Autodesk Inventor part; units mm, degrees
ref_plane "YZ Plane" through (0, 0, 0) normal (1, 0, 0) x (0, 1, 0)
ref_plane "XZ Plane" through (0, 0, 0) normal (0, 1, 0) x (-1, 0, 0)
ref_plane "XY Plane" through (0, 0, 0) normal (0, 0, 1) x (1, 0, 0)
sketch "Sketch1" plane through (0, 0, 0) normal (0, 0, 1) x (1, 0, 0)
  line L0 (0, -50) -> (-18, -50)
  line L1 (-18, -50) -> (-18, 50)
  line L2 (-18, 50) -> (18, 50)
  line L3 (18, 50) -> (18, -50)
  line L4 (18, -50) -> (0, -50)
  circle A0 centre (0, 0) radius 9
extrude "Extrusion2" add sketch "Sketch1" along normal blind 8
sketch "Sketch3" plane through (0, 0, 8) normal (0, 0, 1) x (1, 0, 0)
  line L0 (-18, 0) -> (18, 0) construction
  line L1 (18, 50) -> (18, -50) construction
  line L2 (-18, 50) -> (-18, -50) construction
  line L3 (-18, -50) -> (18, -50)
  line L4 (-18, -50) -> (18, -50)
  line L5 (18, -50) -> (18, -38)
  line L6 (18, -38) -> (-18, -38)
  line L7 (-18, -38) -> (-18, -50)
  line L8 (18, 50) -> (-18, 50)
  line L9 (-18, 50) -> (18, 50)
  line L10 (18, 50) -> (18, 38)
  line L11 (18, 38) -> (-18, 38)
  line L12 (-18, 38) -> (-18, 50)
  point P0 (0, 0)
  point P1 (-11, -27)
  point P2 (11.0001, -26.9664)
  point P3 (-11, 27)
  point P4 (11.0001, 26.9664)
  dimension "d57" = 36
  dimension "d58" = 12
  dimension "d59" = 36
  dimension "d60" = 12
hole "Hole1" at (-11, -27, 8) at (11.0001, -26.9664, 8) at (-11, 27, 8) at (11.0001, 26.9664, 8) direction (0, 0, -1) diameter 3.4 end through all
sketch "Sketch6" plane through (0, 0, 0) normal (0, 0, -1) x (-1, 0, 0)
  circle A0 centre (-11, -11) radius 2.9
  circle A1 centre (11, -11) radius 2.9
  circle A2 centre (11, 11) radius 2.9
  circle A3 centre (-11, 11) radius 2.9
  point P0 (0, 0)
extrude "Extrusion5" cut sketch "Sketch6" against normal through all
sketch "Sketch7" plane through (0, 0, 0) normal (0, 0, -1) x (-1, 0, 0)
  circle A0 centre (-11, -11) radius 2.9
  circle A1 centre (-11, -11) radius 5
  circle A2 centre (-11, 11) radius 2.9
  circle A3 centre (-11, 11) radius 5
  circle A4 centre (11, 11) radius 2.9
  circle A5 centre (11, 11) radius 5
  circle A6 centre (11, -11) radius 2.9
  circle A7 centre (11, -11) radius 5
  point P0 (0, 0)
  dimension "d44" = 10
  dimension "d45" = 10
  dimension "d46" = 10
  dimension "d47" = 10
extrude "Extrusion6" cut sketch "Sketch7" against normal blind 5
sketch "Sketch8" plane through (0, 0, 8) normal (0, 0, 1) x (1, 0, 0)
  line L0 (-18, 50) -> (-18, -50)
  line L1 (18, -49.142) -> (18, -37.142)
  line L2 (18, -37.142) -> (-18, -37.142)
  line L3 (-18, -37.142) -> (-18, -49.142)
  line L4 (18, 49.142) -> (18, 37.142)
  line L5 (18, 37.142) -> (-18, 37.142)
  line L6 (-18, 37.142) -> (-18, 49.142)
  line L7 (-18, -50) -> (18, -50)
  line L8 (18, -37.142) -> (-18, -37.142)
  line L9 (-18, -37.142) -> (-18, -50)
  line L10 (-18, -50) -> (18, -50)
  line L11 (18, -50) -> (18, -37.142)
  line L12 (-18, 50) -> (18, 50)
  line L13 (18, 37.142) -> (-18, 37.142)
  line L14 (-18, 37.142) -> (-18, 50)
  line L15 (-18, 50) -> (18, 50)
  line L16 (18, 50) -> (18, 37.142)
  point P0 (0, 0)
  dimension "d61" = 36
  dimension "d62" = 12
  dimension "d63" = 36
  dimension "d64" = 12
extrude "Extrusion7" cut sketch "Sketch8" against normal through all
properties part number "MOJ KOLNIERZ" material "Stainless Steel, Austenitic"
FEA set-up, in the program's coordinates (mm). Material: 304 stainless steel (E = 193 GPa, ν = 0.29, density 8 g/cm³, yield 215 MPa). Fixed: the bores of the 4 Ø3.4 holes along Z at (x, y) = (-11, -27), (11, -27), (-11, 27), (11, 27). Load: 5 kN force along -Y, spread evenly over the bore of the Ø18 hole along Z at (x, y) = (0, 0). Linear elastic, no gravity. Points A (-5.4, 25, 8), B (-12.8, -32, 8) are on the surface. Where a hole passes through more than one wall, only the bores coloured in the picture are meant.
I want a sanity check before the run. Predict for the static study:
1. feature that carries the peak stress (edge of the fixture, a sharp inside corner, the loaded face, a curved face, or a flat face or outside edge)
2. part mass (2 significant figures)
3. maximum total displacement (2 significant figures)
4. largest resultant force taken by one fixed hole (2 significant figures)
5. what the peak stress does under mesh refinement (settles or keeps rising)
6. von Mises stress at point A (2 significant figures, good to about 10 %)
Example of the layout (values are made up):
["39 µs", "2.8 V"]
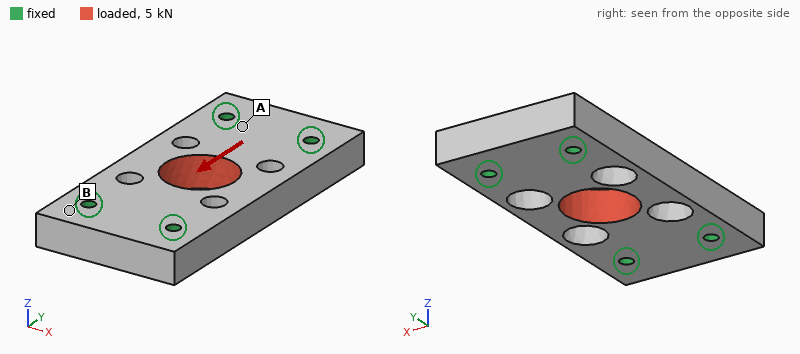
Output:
["a sharp inside corner", "140 g", "3.8 µm", "1.3 kN", "keeps rising", "9.7 MPa"]
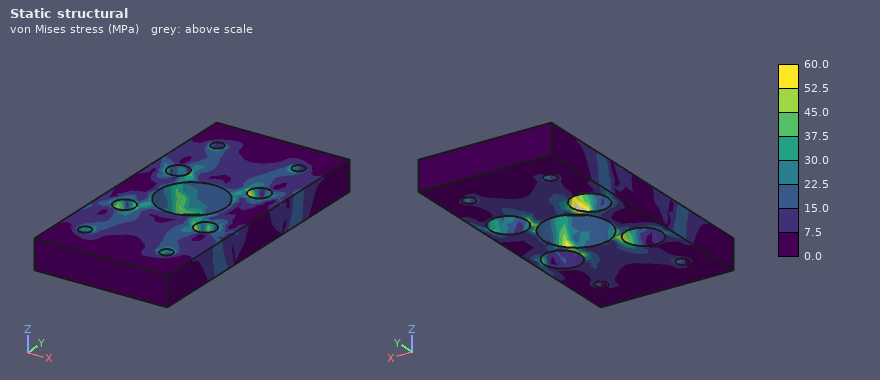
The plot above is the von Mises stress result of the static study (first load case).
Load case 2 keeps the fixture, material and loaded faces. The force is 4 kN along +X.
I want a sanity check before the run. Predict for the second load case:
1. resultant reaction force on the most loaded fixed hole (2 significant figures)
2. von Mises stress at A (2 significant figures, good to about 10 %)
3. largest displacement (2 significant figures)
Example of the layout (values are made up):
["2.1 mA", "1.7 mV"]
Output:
["1.4 kN", "12 MPa", "5.5 µm"]
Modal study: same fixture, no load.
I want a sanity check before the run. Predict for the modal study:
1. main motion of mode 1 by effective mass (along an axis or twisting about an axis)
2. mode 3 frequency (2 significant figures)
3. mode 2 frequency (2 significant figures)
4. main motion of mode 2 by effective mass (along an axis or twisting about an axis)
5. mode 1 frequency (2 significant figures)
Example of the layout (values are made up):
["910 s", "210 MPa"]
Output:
["along Z", "24 kHz", "15 kHz", "twisting about Y", "12 kHz"]
